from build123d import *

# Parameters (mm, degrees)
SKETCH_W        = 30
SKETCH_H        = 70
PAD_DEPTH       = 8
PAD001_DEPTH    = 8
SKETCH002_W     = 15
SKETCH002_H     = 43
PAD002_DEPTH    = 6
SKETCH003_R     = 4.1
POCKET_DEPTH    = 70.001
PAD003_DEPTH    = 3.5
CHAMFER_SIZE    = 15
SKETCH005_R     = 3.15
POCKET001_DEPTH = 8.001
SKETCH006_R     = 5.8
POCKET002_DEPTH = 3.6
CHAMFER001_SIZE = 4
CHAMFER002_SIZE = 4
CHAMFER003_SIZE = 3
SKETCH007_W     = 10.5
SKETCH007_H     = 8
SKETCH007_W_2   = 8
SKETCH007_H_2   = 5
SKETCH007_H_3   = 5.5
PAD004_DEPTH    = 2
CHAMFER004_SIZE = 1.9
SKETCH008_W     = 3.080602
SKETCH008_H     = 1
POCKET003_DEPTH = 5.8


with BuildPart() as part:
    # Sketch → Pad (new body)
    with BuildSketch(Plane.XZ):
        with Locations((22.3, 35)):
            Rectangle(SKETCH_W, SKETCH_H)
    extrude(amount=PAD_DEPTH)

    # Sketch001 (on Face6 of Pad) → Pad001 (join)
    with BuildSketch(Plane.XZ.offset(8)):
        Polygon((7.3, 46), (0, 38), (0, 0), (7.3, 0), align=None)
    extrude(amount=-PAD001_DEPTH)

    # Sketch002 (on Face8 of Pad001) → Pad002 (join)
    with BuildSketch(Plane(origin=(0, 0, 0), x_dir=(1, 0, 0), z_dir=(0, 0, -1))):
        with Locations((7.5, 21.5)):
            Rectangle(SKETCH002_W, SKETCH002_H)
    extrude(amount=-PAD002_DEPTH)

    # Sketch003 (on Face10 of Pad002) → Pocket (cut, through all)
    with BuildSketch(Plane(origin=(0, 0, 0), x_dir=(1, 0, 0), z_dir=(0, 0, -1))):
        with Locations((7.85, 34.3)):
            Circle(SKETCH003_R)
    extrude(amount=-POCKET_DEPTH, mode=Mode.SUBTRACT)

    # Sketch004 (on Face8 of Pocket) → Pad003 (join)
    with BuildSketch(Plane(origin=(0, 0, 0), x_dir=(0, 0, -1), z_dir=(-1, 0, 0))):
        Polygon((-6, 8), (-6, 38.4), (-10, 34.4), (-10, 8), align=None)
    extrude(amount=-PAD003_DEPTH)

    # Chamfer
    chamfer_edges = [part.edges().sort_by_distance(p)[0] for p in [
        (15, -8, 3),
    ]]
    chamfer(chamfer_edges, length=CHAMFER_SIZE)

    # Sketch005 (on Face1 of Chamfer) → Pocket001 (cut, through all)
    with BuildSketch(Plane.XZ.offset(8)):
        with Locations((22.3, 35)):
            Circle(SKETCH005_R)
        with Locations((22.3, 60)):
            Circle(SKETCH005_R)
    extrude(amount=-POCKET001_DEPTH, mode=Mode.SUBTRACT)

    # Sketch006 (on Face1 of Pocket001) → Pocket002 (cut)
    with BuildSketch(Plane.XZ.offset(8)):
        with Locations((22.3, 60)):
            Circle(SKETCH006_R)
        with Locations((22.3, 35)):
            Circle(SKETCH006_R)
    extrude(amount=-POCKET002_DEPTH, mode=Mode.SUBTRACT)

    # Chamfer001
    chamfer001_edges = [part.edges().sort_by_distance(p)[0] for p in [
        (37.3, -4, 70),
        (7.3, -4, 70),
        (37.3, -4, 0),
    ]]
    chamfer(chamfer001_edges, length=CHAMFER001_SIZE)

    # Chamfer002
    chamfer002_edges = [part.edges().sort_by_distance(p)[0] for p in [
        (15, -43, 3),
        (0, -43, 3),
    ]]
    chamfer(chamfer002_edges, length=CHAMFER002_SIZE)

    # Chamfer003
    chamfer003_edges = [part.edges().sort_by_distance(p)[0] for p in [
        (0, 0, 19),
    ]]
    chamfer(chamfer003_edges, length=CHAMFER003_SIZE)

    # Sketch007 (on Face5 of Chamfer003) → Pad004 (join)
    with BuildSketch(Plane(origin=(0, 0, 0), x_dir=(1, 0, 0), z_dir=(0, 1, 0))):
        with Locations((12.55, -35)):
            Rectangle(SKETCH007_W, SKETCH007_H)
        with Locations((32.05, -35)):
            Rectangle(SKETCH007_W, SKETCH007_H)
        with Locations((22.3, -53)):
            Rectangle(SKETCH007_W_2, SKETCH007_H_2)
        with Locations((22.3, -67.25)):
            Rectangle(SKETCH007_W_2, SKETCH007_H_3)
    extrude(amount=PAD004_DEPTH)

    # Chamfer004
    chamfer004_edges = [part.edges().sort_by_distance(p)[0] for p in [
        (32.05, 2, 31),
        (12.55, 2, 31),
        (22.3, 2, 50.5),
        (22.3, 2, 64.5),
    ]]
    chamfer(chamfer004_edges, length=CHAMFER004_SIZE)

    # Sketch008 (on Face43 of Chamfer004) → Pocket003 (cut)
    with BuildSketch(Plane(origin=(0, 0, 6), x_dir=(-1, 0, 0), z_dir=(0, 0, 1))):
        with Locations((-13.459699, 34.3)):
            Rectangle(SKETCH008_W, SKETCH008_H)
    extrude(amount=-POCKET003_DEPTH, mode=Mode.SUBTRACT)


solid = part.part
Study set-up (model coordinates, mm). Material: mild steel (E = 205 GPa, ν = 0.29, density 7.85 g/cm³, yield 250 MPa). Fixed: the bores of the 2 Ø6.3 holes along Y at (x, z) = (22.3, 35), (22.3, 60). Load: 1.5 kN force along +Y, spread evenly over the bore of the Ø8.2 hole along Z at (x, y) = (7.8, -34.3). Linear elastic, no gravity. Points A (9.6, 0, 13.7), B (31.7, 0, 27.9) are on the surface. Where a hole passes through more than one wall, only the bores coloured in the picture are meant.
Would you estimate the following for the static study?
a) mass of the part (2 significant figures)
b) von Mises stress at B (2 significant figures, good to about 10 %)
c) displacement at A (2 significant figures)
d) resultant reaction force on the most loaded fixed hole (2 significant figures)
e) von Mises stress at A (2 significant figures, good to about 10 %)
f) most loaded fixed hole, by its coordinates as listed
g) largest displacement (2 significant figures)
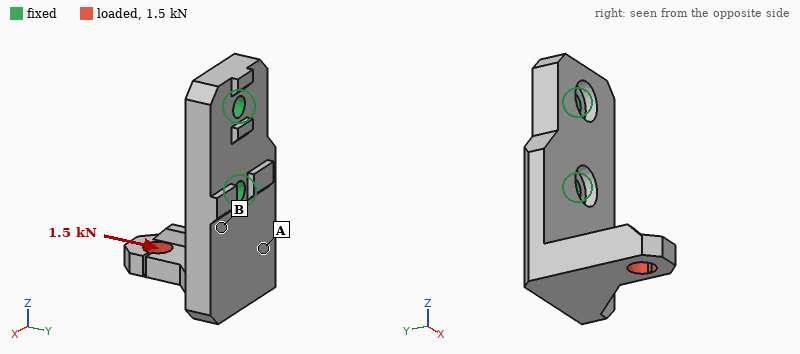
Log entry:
170 g
100 MPa
0.067 mm
3.1 kN
52 MPa
(22.3, 35)
0.20 mm
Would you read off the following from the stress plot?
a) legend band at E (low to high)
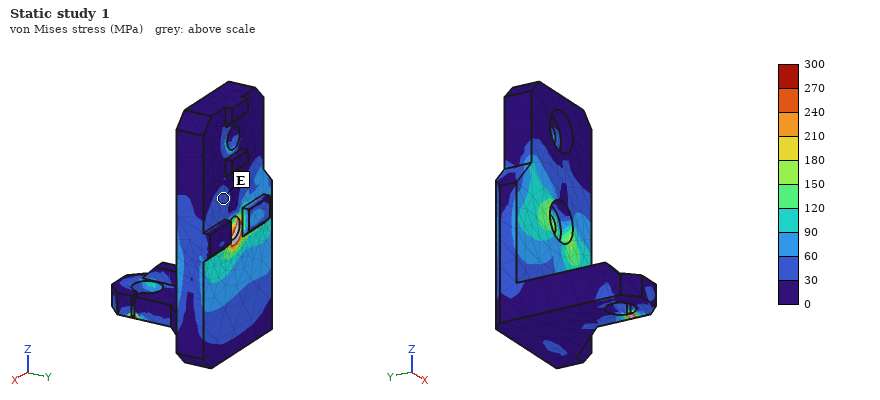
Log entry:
30 to 60 MPa
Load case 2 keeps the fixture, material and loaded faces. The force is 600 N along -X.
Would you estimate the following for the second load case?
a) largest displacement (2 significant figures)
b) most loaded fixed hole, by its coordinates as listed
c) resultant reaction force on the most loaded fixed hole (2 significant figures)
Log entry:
0.10 mm
(22.3, 35)
1.1 kN
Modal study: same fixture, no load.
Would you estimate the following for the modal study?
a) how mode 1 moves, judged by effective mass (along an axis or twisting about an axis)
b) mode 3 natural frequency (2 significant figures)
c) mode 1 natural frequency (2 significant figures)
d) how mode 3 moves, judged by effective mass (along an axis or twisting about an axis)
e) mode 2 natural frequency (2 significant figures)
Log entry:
along Y
5300 Hz
2200 Hz
along Y
3400 Hz
